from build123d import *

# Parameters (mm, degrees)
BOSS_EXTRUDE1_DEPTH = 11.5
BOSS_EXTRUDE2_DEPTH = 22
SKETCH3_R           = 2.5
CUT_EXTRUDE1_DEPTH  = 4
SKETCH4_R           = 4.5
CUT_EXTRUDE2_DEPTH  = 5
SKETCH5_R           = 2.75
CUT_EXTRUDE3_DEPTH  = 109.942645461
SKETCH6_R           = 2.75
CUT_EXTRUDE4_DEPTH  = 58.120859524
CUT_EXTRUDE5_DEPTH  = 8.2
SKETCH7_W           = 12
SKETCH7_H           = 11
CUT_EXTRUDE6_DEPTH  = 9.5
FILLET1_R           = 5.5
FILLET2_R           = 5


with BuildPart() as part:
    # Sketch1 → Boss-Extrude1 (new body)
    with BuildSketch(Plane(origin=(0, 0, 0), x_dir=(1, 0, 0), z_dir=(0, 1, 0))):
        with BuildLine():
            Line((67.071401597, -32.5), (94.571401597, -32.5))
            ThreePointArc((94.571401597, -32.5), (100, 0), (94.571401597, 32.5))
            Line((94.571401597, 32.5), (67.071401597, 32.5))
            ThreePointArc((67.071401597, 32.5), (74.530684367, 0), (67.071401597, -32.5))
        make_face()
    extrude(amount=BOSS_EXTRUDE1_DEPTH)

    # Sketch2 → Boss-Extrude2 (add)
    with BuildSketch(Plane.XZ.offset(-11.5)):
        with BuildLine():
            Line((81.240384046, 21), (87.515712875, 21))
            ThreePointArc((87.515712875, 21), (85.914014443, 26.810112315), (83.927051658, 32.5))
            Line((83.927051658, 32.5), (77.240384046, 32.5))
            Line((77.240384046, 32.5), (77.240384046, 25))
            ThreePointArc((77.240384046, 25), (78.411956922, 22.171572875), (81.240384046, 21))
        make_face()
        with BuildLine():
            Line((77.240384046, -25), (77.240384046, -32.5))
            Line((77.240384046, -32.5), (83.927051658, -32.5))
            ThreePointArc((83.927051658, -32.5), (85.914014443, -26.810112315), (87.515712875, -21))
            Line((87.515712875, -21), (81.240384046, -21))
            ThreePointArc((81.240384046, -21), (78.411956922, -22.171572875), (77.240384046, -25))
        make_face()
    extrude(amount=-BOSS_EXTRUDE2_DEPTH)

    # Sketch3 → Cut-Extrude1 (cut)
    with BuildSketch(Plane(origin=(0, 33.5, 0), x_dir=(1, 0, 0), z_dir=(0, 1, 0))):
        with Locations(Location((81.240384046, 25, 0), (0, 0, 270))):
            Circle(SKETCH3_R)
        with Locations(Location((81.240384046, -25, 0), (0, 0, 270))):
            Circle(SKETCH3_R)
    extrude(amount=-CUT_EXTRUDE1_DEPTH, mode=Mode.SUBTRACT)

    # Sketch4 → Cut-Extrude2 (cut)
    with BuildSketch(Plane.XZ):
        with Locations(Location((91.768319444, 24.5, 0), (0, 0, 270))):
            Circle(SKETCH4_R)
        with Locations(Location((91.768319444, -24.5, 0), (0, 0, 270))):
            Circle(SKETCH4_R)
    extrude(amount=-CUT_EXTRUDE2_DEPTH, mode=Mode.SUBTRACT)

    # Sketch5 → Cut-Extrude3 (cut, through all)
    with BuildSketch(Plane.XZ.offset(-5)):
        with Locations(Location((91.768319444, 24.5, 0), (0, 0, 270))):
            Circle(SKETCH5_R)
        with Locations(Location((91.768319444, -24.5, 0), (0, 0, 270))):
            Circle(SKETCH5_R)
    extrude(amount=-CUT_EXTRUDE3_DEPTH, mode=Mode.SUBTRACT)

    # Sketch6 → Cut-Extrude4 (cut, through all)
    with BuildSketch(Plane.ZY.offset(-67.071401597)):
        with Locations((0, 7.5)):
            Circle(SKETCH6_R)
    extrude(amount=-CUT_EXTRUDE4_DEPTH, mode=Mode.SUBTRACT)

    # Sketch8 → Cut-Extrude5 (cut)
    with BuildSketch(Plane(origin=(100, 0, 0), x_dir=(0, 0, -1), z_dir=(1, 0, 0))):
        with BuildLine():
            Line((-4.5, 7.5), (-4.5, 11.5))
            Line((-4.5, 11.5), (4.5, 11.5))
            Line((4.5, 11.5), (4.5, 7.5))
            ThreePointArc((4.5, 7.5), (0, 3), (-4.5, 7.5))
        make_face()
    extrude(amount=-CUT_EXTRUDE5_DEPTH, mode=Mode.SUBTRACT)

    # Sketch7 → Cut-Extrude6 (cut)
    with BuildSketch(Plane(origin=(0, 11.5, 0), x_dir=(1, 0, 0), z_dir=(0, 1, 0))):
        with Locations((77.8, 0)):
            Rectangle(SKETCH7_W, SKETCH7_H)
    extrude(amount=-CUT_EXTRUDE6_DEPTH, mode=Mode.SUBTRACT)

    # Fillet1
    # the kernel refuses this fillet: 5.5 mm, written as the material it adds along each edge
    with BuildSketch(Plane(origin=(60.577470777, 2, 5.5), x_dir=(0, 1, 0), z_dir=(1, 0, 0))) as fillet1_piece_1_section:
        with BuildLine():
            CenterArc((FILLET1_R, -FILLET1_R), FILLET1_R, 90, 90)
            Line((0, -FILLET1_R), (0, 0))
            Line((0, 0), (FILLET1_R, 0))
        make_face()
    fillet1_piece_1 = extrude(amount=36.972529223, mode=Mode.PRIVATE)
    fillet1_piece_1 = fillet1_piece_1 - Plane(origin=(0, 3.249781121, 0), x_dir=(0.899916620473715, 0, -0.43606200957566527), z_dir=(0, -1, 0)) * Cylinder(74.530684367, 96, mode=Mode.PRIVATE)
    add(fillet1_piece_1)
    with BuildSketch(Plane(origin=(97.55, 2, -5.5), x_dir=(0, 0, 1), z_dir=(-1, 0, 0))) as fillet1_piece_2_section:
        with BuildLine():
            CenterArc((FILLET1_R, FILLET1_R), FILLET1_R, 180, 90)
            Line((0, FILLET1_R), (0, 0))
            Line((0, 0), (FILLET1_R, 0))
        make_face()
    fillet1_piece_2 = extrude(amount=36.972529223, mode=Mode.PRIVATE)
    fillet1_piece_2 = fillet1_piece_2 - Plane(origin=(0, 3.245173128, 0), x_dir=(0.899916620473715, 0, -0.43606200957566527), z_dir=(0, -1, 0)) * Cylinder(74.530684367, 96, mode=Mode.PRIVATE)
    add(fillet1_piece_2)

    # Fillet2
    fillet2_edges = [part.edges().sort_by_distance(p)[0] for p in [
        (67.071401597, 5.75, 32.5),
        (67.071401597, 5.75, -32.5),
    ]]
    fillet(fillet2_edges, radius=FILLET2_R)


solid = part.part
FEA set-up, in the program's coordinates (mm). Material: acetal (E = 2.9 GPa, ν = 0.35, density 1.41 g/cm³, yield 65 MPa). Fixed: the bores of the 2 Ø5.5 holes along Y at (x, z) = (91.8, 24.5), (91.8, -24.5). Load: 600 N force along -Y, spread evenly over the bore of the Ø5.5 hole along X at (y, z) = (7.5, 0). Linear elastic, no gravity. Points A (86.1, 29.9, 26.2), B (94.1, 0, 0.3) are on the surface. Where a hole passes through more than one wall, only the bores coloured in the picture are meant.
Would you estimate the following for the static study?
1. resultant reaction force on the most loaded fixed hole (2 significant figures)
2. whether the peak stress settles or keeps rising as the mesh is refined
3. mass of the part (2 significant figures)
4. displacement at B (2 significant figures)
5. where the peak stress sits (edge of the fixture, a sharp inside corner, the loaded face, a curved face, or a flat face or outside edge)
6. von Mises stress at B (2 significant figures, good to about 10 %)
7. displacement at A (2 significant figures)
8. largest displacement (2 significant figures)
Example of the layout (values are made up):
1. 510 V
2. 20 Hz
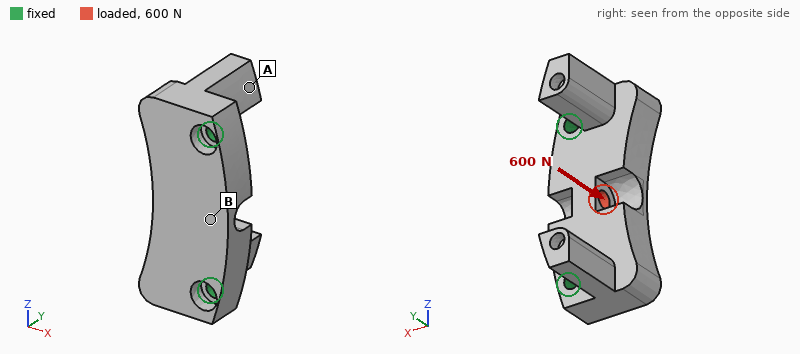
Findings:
1. 440 N
2. keeps rising
3. 29 g
4. 0.12 mm
5. edge of the fixture
6. 11 MPa
7. 0.12 mm
8. 0.17 mm
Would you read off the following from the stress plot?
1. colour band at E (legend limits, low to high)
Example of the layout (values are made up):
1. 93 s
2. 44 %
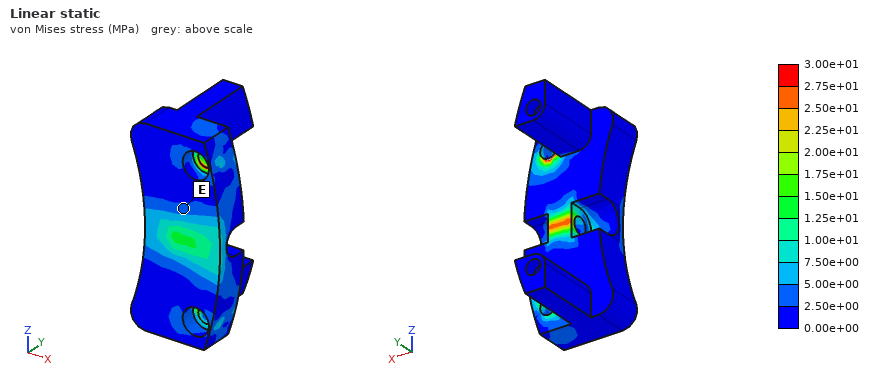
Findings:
1. 2.50e+00 to 5.00e+00 MPa
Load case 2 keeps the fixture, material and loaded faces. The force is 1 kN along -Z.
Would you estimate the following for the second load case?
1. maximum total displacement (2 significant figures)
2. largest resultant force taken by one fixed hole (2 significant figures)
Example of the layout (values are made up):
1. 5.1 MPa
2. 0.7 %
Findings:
1. 49 µm
2. 500 N
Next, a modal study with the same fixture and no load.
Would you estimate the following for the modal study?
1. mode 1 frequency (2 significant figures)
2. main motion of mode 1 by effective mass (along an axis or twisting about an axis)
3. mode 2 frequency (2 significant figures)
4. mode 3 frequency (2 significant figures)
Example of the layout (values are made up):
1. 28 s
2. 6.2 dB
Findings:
1. 1900 Hz
2. along Y
3. 2300 Hz
4. 2600 Hz
